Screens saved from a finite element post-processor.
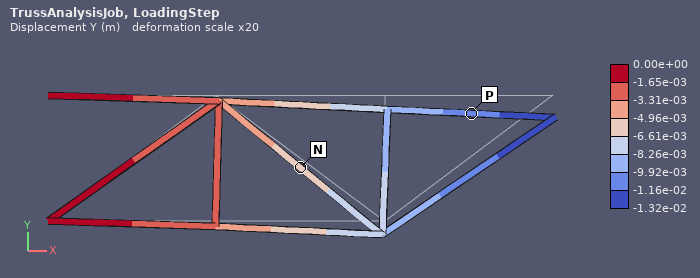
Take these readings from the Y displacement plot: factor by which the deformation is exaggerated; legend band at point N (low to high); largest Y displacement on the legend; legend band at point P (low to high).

20
-6.61e-03 to -4.96e-03 m
0.00e+00 m
-1.16e-02 to -9.92e-03 m
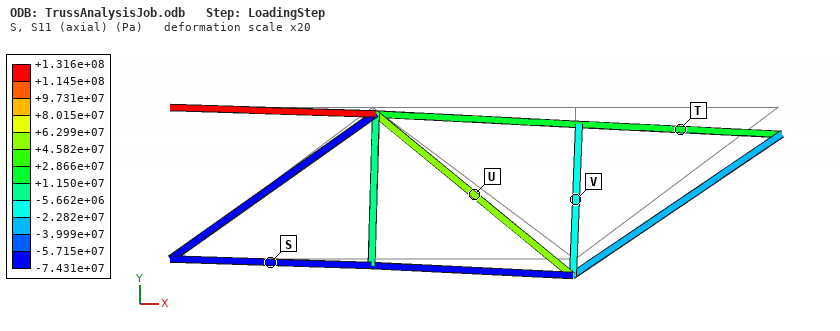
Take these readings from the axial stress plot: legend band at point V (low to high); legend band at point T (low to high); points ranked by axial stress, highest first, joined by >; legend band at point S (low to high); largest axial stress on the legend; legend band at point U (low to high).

-2.282e+07 to -5.662e+06 Pa
+1.150e+07 to +2.866e+07 Pa
U > T > V > S
-7.431e+07 to -5.715e+07 Pa
+1.316e+08 Pa
+4.582e+07 to +6.299e+07 Pa
